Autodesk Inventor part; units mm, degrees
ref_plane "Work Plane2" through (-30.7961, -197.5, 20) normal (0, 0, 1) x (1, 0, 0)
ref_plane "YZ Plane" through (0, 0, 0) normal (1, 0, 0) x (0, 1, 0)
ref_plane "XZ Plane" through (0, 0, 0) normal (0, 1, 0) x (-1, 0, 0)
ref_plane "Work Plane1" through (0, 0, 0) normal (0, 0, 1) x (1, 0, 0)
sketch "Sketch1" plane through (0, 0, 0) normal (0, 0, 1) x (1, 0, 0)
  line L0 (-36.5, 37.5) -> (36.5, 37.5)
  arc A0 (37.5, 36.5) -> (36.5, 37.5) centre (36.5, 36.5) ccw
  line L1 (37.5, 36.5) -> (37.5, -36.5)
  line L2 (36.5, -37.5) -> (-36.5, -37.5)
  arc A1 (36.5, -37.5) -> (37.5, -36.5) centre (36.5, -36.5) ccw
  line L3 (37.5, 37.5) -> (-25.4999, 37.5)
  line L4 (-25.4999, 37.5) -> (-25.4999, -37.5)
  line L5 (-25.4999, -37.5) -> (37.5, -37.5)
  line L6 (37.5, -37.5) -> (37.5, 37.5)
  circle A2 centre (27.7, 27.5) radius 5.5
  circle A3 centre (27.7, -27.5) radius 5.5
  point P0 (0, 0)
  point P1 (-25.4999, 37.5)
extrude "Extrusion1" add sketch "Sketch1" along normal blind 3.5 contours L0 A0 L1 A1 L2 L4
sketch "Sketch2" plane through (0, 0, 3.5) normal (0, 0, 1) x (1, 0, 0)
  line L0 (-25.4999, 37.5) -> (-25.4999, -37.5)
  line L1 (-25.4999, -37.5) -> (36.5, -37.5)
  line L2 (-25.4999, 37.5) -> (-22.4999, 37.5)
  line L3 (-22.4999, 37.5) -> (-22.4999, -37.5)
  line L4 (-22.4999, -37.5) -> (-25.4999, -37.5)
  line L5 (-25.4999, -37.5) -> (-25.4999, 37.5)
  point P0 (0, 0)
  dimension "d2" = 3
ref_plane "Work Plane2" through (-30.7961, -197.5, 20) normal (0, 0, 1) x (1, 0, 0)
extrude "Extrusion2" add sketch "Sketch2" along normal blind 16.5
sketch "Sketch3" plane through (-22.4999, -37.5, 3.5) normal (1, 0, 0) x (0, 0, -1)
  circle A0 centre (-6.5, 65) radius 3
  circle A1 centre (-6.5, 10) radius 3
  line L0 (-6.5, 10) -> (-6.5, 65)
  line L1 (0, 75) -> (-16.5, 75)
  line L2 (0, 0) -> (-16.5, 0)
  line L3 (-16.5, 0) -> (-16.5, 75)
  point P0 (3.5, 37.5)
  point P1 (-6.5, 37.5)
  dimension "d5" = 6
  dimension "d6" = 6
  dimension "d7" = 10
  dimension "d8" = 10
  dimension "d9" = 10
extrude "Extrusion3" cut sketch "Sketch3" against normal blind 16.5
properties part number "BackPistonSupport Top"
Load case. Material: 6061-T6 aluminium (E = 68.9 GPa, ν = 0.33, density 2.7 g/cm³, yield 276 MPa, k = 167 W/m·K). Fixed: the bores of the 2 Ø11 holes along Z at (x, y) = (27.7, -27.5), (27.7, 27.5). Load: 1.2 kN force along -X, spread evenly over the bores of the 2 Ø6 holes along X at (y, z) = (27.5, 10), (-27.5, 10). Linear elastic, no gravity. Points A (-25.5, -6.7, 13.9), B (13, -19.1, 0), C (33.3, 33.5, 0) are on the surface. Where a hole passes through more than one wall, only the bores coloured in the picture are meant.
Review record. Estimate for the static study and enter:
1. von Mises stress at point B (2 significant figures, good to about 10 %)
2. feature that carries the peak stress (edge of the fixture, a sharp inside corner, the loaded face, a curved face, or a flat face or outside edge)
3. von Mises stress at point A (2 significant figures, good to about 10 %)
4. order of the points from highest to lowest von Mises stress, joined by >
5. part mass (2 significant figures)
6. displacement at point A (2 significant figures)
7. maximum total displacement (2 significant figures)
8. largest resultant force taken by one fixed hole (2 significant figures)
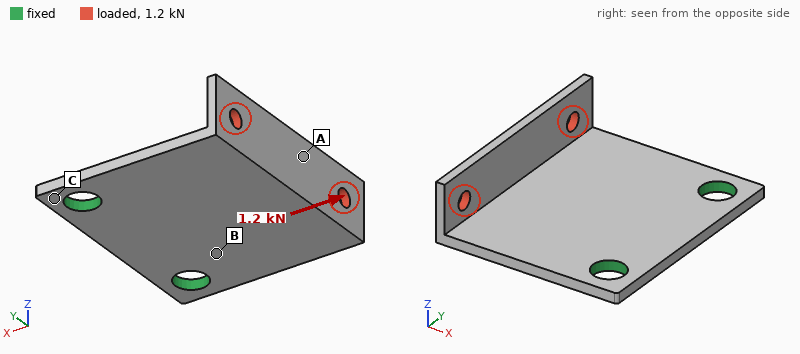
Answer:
55 MPa
a flat face or outside edge
26 MPa
B > A > C
52 g
0.74 mm
0.88 mm
610 N
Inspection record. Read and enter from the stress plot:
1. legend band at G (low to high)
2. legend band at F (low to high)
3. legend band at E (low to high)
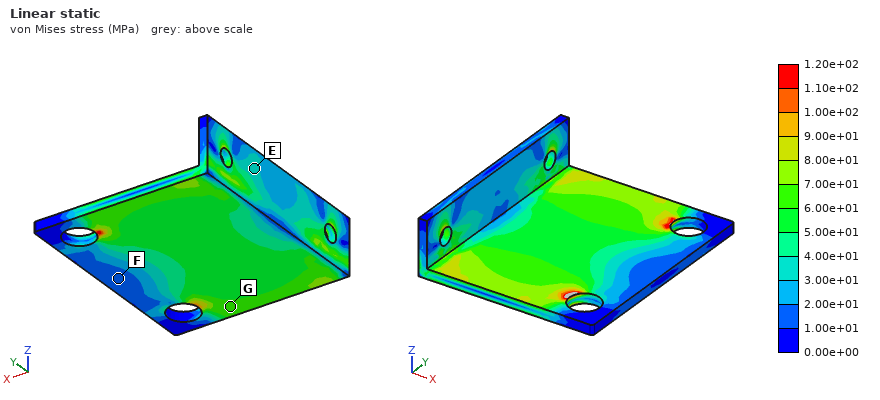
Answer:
6.00e+01 to 7.00e+01 MPa
1.00e+01 to 2.00e+01 MPa
3.00e+01 to 4.00e+01 MPa
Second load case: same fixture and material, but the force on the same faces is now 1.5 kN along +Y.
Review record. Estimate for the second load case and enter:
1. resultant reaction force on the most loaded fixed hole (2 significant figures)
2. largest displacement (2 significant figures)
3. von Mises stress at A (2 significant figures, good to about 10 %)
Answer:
1.5 kN
0.51 mm
26 MPa
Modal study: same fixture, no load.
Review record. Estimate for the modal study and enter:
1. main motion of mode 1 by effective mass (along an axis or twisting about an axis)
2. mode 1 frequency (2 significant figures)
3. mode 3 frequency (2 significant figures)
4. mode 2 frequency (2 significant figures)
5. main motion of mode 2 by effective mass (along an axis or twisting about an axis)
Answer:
along Z
770 Hz
3900 Hz
1600 Hz
twisting about X
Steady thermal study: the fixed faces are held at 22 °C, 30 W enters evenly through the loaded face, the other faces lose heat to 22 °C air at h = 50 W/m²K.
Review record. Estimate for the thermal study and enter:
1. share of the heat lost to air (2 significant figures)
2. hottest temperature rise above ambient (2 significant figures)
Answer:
33 %
40 K
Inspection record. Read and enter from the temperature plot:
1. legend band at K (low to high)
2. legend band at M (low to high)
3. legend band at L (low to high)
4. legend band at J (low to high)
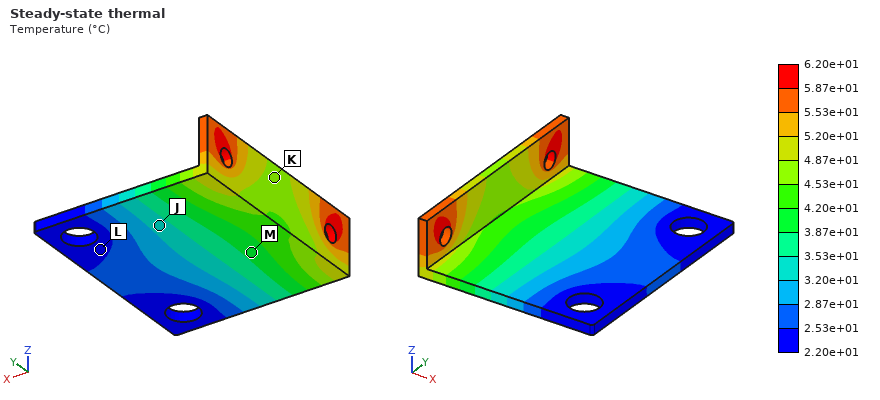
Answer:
4.53e+01 to 4.87e+01 °C
3.87e+01 to 4.20e+01 °C
2.20e+01 to 2.53e+01 °C
3.20e+01 to 3.53e+01 °C
